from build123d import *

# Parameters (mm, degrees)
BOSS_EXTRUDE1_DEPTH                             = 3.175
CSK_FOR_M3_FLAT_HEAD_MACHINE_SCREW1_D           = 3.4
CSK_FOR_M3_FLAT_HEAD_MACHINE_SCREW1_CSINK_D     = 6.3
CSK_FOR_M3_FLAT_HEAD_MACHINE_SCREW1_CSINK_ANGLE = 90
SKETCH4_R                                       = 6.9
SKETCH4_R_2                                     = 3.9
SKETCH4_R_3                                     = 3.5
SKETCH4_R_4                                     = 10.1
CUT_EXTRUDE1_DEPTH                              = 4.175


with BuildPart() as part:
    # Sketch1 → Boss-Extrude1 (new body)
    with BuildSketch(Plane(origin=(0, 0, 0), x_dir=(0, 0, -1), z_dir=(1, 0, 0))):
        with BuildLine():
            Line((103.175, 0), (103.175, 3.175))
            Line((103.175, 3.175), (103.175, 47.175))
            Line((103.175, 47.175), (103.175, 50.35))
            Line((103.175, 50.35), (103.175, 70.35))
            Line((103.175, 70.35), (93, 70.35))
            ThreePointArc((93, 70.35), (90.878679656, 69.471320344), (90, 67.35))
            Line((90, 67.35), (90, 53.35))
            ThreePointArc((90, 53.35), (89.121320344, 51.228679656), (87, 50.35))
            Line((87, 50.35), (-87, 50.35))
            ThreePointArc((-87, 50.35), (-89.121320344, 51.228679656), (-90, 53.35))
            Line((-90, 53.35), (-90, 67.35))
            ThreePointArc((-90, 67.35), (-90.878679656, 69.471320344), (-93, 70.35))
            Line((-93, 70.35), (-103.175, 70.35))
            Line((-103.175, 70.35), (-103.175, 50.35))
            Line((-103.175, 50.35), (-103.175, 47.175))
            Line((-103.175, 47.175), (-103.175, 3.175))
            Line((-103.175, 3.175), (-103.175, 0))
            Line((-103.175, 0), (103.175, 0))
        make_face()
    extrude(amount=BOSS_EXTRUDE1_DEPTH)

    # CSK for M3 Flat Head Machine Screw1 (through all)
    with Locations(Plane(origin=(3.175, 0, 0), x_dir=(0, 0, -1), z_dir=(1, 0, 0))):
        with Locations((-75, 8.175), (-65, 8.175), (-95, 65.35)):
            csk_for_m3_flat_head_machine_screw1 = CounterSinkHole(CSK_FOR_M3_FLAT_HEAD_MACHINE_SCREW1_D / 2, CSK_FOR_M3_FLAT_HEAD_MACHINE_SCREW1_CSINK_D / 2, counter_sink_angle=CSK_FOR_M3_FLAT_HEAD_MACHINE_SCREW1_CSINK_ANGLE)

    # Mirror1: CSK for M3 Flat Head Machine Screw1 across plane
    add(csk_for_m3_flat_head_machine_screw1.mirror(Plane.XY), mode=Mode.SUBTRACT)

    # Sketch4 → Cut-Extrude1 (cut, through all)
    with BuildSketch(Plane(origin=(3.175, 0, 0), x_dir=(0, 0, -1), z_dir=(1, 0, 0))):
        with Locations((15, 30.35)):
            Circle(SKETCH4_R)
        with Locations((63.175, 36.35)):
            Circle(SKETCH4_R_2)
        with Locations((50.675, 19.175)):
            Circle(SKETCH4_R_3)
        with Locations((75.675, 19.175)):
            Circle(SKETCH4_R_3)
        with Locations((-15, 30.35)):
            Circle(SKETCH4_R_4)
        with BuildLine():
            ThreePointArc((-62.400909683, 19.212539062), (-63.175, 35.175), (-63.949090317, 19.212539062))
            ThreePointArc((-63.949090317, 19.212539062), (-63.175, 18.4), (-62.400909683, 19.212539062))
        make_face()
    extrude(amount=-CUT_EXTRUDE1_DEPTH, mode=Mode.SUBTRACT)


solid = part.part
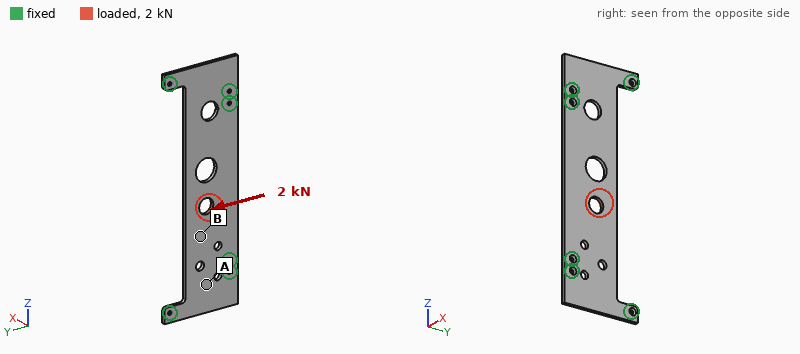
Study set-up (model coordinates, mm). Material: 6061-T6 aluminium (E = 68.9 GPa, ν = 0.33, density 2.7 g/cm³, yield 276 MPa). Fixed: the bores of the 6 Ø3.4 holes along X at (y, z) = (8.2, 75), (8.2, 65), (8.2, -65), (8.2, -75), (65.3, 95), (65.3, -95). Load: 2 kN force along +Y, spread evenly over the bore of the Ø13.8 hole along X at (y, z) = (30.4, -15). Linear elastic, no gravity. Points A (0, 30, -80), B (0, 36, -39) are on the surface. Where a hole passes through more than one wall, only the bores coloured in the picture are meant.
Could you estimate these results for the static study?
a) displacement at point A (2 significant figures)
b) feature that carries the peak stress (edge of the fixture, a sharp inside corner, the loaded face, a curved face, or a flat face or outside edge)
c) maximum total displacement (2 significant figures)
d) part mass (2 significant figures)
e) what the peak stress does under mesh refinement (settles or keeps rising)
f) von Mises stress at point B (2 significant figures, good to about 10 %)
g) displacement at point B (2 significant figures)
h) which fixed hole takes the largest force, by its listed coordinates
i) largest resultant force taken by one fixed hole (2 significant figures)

8.1 µm
edge of the fixture
52 µm
86 g
keeps rising
18 MPa
34 µm
(8.2, -65)
1.4 kN
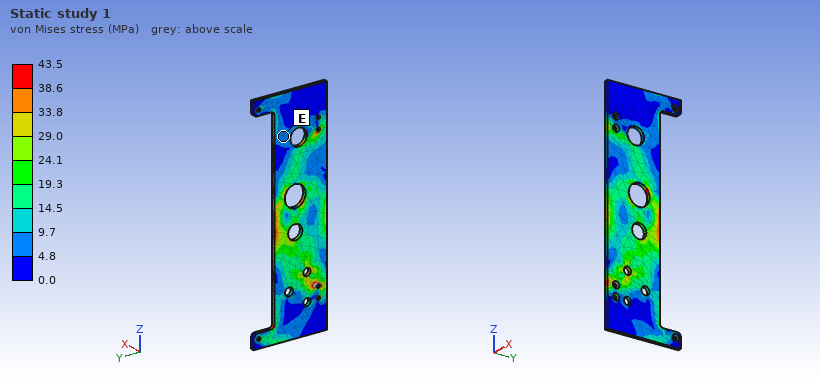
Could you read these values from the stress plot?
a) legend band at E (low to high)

4.8 to 9.7 MPa
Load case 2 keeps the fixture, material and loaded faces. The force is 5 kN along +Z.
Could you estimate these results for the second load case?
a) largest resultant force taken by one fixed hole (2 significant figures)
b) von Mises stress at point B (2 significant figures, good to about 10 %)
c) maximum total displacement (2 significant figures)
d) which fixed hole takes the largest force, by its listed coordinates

1.6 kN
23 MPa
38 µm
(8.2, -65)
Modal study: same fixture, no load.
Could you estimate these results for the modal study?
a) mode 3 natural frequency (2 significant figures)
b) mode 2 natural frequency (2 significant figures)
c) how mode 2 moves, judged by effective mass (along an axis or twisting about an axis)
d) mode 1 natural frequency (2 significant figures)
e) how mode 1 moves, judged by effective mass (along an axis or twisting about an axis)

1600 Hz
1400 Hz
twisting about Z
680 Hz
along X
